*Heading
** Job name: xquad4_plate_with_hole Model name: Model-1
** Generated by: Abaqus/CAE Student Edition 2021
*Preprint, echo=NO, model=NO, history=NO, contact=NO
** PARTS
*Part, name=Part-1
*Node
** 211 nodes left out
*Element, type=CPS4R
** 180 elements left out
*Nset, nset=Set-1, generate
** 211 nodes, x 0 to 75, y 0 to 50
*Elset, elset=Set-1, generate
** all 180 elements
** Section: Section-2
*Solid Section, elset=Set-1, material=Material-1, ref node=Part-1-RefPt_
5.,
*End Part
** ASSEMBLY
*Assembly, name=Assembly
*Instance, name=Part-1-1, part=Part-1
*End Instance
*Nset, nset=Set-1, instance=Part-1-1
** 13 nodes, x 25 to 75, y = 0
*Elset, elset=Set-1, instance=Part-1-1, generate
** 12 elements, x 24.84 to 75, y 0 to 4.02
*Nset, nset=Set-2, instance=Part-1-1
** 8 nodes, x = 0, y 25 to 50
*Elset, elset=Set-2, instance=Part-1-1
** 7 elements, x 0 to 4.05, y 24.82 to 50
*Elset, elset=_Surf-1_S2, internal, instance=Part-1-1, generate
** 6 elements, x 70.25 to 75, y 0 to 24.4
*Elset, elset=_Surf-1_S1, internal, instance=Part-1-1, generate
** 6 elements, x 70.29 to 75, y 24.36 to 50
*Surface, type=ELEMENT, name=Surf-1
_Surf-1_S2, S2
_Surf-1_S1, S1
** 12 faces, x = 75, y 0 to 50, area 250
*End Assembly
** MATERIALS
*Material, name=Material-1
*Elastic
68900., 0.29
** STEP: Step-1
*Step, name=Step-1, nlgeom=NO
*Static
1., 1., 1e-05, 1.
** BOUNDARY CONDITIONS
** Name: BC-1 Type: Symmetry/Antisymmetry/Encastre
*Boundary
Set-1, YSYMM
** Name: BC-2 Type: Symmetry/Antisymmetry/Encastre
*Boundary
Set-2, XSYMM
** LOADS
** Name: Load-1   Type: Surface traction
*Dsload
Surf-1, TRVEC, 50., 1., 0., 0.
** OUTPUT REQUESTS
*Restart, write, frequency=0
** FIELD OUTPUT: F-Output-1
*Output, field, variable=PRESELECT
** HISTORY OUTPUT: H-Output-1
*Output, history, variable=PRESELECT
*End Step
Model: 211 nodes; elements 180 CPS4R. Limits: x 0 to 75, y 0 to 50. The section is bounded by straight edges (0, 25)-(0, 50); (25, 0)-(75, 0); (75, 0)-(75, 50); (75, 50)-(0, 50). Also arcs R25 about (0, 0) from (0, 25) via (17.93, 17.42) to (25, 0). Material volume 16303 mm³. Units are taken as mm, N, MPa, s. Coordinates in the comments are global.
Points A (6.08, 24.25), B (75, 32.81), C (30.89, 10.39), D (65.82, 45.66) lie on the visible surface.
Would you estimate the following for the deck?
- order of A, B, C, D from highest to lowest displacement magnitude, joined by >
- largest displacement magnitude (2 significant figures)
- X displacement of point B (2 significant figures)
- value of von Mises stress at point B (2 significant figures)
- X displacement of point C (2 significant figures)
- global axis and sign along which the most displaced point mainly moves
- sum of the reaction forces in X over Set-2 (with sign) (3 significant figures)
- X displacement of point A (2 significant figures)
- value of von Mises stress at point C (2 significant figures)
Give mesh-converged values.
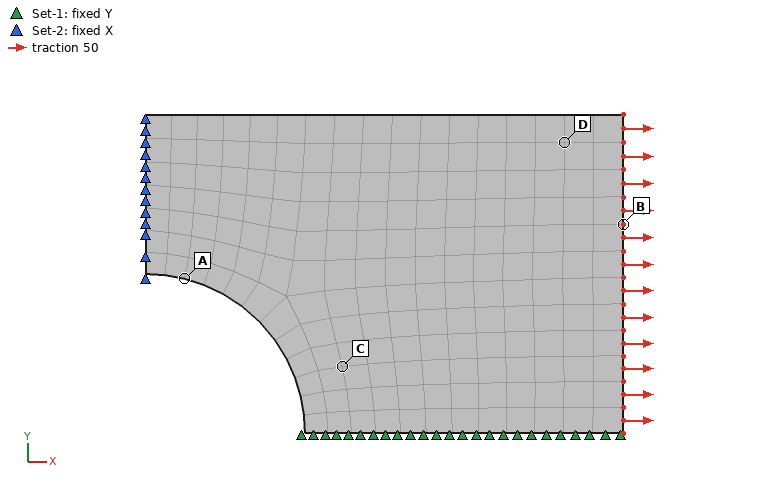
B > C > D > A
0.10 mm
0.081 mm
46 MPa
0.076 mm
+X
-12500 N
0.020 mm
47 MPa
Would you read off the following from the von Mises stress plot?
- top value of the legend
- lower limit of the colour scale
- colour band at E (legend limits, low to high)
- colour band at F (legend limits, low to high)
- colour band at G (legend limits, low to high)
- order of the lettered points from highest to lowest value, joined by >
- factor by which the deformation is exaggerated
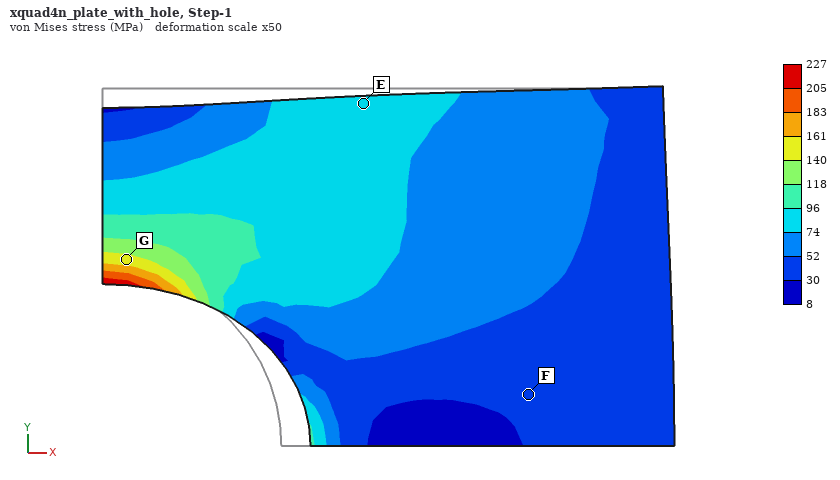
227 MPa
8 MPa
74 to 96 MPa
30 to 52 MPa
140 to 161 MPa
G > E > F
50
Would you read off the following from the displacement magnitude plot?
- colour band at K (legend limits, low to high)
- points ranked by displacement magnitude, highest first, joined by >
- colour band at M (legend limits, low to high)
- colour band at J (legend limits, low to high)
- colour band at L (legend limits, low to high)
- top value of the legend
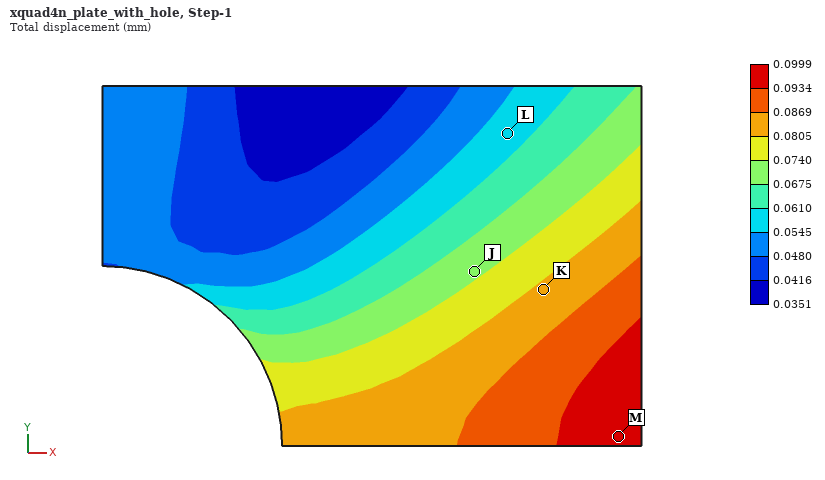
0.0805 to 0.0869 mm
M > K > J > L
0.0934 to 0.0999 mm
0.0675 to 0.0740 mm
0.0545 to 0.0610 mm
0.0999 mm
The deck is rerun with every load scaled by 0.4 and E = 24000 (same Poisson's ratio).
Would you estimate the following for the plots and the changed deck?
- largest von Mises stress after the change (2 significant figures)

91 MPa
